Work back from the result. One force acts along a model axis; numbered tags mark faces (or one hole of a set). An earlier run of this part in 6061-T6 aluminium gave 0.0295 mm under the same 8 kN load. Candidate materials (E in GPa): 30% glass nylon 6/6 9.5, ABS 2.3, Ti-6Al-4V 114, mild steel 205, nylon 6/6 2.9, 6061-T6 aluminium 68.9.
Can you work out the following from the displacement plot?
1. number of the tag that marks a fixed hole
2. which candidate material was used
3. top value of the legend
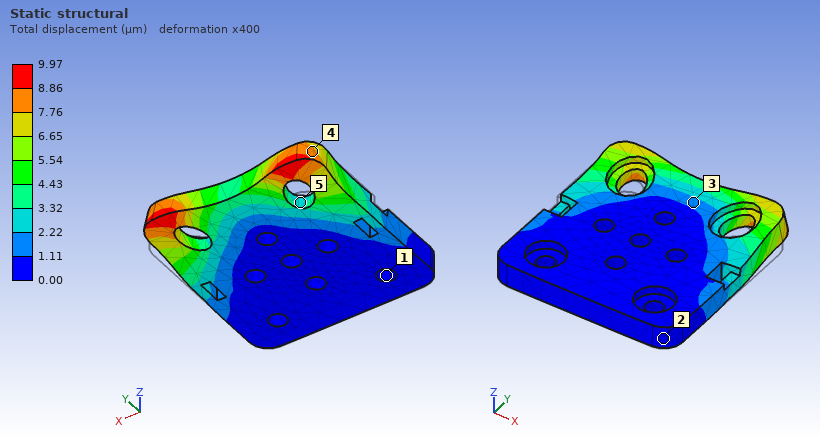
1
mild steel
9.97 µm
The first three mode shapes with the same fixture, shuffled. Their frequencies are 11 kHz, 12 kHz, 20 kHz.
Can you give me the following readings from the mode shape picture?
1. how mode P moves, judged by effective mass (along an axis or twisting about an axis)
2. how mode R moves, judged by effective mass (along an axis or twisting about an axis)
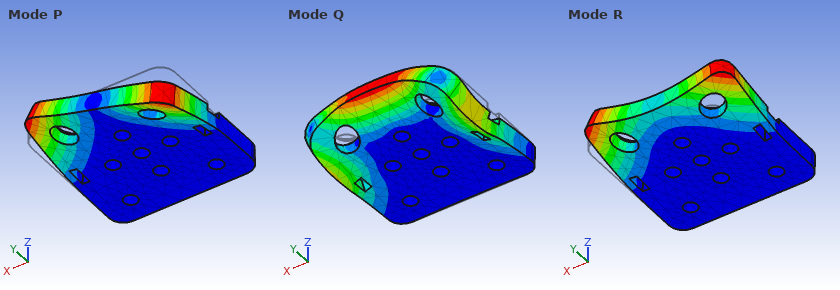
twisting about Y
along Z
